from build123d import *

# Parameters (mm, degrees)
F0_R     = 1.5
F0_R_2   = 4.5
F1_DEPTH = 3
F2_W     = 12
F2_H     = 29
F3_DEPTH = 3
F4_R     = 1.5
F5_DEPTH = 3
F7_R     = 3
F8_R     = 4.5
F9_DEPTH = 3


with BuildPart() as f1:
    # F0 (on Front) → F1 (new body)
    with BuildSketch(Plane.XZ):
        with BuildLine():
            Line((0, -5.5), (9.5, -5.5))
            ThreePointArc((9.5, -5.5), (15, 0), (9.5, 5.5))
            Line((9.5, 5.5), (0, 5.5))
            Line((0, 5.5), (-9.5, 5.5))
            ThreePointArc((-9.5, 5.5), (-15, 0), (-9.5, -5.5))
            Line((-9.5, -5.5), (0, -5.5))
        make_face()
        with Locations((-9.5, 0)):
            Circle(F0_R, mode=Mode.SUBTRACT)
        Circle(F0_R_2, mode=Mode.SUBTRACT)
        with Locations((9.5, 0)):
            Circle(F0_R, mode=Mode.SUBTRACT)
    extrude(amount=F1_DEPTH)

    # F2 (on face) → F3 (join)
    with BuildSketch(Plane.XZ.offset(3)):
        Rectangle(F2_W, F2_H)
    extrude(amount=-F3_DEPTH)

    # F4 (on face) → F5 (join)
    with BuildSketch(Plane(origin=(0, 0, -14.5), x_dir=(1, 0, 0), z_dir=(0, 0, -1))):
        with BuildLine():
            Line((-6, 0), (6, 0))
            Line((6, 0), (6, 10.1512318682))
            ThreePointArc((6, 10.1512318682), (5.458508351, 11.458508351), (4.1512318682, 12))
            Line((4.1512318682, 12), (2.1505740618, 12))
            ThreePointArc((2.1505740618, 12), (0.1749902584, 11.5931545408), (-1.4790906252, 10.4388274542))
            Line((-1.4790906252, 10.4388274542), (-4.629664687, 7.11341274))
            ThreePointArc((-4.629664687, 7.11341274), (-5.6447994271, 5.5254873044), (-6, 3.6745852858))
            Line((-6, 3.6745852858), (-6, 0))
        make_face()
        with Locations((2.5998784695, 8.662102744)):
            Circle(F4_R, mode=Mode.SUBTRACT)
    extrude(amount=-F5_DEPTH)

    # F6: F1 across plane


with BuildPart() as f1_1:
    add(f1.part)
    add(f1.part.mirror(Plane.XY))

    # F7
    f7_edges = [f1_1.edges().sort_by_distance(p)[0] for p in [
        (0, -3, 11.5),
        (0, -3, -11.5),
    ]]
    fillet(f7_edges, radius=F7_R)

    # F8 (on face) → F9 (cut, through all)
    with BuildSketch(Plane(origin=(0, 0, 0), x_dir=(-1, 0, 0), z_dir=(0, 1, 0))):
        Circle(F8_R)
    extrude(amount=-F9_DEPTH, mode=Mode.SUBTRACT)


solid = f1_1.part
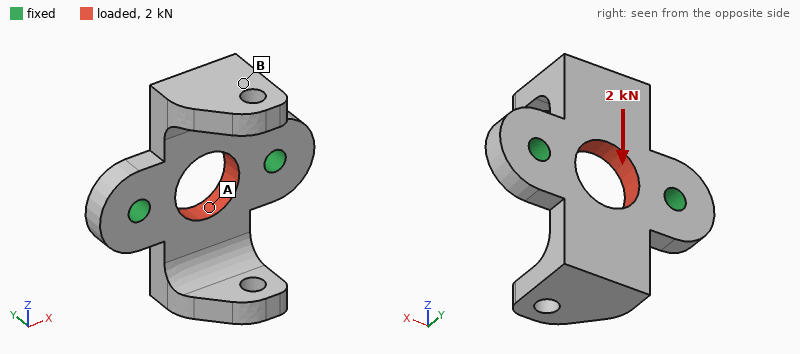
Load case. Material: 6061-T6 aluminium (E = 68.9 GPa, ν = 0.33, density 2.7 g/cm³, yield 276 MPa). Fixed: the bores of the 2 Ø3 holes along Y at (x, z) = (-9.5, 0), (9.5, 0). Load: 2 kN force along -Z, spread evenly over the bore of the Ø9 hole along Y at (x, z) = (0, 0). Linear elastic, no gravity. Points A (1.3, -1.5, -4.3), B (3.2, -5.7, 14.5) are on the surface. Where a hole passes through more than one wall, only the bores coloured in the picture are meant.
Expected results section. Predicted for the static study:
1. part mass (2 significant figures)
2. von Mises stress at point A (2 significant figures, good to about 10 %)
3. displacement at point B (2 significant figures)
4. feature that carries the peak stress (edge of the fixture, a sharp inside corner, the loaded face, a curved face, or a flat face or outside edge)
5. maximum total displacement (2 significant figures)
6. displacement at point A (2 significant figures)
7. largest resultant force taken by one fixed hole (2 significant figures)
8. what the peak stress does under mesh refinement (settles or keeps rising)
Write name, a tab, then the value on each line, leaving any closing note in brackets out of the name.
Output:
part mass	5.0 g
von Mises stress at point A	39 MPa
displacement at point B	7.3 µm
feature that carries the peak stress	edge of the fixture
maximum total displacement	8.7 µm
displacement at point A	8.7 µm
largest resultant force taken by one fixed hole	1.0 kN
what the peak stress does under mesh refinement	keeps rising
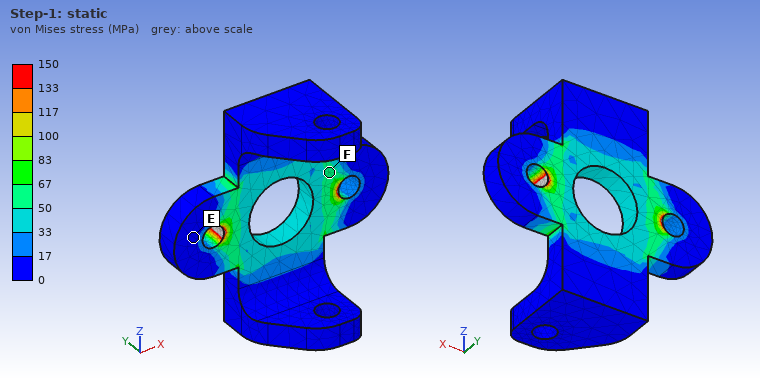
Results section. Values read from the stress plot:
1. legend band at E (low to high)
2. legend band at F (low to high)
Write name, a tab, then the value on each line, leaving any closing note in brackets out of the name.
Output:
legend band at E	0 to 17 MPa
legend band at F	50 to 67 MPa
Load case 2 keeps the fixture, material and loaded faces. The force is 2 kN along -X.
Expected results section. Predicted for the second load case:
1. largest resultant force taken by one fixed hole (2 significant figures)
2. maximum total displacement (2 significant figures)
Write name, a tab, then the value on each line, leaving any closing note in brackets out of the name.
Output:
largest resultant force taken by one fixed hole	1.0 kN
maximum total displacement	5.6 µm
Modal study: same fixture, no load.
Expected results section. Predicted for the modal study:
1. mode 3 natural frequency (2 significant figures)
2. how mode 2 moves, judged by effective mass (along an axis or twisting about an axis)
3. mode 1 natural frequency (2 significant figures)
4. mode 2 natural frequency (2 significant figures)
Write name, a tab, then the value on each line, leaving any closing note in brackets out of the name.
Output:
mode 3 natural frequency	15 kHz
how mode 2 moves, judged by effective mass	along Y
mode 1 natural frequency	5700 Hz
mode 2 natural frequency	6000 Hz
